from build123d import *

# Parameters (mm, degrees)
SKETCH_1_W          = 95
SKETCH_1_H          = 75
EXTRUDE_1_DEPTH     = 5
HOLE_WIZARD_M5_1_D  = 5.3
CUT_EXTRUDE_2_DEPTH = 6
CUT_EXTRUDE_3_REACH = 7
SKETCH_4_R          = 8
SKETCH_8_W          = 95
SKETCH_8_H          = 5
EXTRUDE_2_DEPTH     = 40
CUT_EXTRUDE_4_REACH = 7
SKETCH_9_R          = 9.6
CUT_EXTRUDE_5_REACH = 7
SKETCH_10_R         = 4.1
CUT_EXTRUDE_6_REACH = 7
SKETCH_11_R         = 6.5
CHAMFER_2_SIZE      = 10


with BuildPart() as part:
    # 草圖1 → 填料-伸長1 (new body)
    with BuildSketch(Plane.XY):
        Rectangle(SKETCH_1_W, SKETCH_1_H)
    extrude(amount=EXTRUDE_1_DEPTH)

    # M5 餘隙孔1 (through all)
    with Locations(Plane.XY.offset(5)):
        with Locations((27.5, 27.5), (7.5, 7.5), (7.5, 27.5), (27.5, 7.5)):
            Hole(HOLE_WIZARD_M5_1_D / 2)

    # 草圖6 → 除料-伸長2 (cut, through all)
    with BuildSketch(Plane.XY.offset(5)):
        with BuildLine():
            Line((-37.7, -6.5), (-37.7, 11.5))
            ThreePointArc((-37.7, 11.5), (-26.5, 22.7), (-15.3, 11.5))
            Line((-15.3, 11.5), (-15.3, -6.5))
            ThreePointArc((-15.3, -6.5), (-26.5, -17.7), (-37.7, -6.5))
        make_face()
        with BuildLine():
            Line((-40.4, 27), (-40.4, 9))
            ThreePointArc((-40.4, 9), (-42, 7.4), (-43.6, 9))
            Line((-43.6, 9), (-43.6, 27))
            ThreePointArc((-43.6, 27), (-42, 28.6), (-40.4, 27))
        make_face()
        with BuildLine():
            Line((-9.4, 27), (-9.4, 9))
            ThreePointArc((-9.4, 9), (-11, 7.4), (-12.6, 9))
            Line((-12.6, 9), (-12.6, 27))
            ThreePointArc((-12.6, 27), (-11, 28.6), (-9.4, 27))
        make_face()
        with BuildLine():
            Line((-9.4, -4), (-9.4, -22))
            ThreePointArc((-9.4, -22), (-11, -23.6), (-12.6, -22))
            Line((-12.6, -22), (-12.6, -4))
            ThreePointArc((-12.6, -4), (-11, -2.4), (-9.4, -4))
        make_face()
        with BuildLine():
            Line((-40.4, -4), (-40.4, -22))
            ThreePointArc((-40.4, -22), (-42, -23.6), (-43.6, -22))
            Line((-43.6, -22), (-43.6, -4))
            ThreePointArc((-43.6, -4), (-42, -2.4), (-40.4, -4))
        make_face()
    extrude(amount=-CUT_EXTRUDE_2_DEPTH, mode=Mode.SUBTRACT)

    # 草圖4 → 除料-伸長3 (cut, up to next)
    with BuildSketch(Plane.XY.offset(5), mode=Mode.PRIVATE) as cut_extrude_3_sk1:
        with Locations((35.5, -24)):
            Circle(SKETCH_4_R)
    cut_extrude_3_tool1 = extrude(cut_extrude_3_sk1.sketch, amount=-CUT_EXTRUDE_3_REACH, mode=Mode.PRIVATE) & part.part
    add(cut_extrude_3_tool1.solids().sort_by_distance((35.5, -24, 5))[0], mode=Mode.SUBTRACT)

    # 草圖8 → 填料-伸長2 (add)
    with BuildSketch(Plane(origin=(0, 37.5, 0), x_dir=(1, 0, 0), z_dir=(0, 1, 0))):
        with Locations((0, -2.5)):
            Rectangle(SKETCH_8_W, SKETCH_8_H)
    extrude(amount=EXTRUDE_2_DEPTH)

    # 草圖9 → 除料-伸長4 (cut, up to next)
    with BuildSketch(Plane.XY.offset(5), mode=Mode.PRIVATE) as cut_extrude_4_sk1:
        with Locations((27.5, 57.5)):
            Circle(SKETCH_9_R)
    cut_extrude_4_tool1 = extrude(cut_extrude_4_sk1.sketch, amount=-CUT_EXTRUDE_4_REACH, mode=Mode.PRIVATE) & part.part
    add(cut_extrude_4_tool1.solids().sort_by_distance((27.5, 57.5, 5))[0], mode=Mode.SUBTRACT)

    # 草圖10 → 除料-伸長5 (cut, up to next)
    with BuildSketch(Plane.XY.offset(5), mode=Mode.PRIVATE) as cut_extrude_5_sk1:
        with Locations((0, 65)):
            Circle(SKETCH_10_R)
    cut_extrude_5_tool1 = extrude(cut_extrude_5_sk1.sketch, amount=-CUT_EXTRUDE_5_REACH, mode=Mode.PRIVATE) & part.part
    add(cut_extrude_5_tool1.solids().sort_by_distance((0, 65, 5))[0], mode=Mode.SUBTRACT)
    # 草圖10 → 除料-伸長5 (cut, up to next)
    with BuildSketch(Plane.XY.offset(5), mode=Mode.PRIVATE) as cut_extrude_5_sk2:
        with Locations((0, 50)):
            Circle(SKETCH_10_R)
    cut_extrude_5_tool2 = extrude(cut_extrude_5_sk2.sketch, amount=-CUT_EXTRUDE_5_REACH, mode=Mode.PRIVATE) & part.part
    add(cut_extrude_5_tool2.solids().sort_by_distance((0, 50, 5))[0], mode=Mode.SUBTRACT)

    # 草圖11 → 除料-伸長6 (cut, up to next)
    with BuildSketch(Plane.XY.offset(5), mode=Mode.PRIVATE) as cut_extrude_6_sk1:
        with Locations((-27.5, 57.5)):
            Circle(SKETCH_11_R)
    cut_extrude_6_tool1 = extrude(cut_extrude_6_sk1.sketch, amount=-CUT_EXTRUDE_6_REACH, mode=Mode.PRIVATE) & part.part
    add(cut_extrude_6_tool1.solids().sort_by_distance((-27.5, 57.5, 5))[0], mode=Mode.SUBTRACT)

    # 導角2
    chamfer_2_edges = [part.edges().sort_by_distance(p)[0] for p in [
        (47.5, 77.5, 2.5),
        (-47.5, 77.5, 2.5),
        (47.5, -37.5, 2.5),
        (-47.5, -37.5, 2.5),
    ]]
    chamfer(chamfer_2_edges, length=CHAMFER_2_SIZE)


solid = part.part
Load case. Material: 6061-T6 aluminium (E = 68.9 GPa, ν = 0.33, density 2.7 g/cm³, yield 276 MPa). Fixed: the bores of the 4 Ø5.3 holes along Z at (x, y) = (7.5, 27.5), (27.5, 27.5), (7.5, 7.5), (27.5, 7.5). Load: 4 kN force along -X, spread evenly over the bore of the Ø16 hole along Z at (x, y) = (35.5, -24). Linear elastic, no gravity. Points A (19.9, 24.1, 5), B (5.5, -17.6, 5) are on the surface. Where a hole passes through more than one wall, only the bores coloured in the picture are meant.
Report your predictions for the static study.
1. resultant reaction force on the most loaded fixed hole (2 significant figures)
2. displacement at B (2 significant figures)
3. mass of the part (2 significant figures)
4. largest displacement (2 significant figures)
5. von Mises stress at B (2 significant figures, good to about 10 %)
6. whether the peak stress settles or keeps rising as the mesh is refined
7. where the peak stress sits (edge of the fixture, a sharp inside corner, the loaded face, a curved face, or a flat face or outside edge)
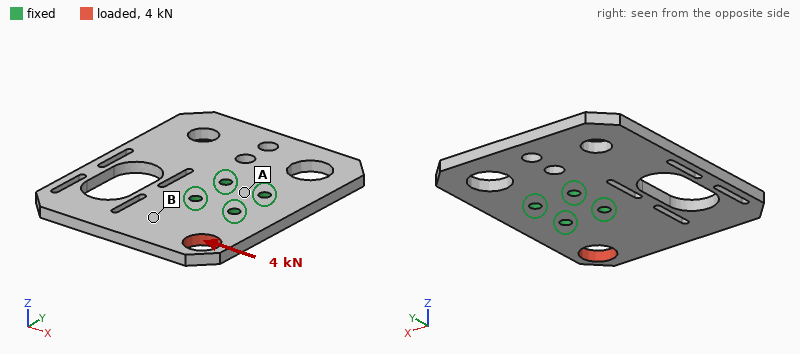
3.8 kN
28 µm
120 g
71 µm
23 MPa
keeps rising
edge of the fixture
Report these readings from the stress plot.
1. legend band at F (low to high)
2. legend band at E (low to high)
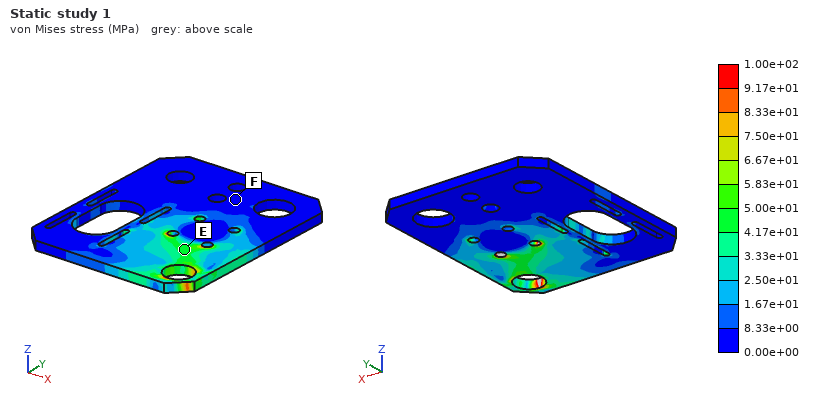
0.00e+00 to 8.33e+00 MPa
4.17e+01 to 5.00e+01 MPa
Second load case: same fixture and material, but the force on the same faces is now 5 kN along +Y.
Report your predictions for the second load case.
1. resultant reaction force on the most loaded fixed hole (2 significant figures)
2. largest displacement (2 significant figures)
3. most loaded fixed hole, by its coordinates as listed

3.8 kN
58 µm
(27.5, 7.5)
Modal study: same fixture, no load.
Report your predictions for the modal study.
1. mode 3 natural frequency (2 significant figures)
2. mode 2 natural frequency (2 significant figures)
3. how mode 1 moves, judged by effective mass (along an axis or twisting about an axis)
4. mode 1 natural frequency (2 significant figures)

1800 Hz
1200 Hz
along Z
1000 Hz
